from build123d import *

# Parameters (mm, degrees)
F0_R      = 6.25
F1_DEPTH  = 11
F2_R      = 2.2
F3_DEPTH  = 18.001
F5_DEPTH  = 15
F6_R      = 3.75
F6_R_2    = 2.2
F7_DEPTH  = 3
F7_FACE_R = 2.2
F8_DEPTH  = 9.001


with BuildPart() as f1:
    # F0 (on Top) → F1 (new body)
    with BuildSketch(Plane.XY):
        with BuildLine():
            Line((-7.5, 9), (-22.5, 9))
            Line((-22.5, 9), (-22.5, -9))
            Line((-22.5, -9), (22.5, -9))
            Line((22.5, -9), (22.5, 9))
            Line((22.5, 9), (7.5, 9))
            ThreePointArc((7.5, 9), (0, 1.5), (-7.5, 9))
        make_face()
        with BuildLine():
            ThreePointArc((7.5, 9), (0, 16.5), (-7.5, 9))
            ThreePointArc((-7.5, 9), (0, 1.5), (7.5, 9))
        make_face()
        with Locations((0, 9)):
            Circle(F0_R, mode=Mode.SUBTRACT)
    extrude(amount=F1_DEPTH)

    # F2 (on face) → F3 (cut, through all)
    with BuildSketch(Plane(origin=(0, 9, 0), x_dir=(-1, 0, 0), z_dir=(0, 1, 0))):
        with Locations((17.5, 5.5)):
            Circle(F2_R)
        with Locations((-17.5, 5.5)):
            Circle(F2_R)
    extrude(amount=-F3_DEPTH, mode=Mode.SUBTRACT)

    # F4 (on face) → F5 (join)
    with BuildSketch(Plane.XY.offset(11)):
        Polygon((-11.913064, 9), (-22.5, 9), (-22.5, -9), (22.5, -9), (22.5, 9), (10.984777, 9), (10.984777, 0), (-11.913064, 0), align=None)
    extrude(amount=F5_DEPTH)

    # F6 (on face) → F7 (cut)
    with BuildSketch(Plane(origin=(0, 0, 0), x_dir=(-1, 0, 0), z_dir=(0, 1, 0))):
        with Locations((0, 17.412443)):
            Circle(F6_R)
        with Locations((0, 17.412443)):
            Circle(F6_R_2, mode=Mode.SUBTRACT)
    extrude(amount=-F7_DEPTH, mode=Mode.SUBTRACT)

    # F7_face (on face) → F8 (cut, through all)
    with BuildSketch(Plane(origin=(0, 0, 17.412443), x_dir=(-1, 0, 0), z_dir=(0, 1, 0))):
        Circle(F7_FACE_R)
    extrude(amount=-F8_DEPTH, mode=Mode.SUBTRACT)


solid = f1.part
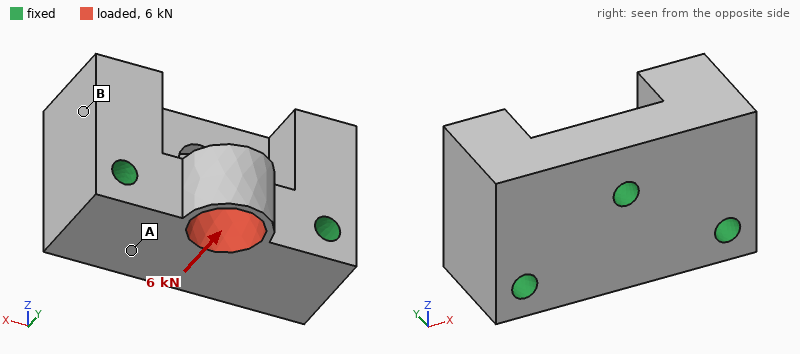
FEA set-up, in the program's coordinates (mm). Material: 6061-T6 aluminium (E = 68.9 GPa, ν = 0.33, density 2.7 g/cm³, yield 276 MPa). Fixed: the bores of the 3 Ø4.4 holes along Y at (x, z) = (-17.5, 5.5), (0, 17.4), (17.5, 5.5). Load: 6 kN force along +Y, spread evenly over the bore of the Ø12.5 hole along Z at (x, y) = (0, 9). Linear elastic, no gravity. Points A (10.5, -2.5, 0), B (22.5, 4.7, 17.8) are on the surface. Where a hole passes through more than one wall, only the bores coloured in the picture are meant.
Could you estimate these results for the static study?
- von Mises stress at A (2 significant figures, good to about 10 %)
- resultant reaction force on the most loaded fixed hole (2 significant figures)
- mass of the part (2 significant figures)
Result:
32 MPa
2.5 kN
45 g
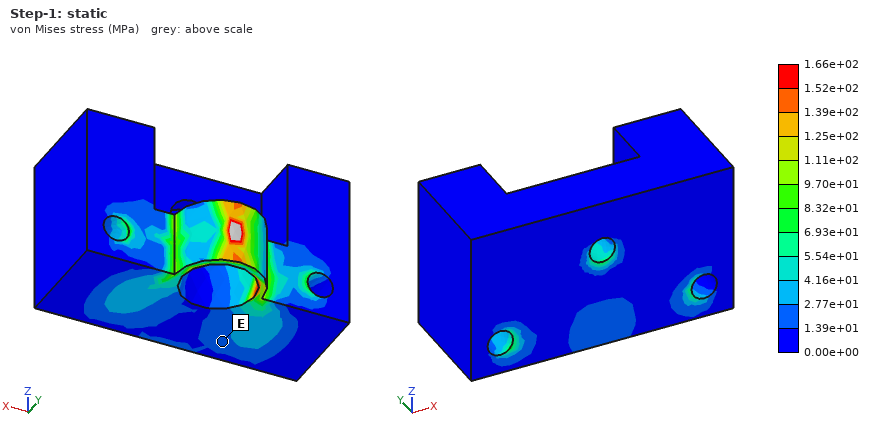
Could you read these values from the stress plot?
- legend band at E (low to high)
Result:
1.39e+01 to 2.77e+01 MPa
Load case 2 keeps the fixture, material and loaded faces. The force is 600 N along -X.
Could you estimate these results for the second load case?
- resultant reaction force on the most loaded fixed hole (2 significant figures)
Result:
300 N
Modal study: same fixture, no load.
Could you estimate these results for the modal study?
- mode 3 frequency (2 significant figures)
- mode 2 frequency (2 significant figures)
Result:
26 kHz
26 kHz
